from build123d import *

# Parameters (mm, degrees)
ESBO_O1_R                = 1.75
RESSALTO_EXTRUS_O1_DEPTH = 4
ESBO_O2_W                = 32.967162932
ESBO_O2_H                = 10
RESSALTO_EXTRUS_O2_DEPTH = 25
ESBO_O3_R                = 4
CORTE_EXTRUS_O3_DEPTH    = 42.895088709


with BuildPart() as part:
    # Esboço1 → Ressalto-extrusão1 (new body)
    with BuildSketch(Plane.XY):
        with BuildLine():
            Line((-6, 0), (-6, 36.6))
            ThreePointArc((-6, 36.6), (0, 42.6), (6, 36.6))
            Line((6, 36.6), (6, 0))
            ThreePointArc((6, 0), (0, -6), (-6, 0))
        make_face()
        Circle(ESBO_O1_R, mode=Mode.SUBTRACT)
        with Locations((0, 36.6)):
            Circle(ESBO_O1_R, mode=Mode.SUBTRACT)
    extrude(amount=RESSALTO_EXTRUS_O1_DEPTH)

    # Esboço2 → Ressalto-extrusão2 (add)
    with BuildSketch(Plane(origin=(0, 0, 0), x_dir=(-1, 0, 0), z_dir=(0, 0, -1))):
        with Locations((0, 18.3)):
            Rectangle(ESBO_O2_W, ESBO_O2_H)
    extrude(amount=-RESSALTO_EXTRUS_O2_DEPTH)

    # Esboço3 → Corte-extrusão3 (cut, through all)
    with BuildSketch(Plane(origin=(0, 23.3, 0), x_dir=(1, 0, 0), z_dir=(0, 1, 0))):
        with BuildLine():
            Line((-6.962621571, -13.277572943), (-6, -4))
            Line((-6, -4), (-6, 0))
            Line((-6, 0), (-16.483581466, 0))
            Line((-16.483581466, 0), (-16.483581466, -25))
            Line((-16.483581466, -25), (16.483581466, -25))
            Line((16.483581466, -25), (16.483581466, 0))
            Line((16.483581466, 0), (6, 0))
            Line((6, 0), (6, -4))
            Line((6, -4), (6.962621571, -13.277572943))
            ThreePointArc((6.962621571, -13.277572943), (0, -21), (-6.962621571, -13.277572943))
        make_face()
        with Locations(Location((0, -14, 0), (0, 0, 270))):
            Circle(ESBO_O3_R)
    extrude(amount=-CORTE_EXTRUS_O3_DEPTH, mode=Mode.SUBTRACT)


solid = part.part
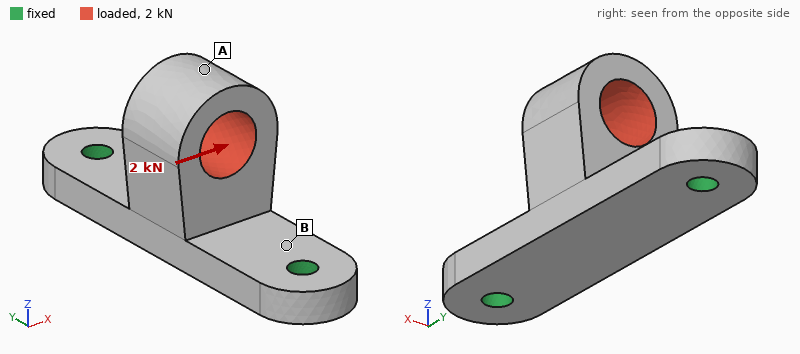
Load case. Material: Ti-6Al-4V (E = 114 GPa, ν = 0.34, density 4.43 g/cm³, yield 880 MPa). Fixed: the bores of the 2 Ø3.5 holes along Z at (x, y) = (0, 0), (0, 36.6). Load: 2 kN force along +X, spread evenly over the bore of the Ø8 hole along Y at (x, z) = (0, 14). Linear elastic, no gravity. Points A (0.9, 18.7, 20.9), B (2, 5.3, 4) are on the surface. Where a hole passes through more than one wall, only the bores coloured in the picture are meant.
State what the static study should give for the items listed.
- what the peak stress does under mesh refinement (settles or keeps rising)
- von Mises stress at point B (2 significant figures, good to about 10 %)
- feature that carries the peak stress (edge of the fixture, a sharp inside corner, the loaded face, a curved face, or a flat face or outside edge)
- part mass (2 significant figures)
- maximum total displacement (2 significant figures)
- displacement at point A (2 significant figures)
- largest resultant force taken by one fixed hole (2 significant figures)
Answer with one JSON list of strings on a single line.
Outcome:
["keeps rising", "380 MPa", "edge of the fixture", "16 g", "0.36 mm", "0.36 mm", "1.0 kN"]
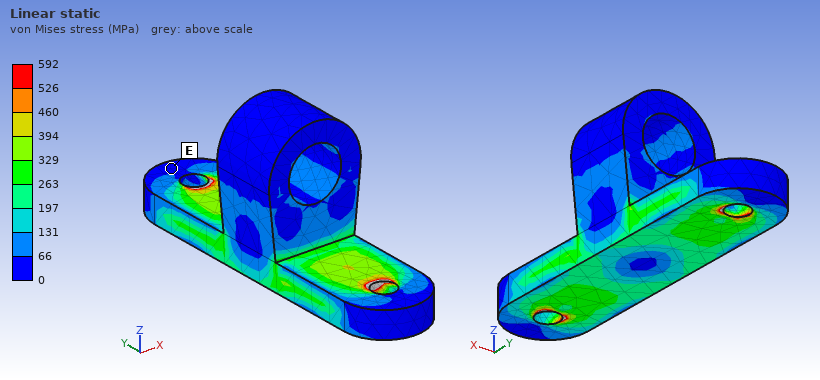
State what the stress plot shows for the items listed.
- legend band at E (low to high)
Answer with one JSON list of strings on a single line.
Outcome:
["0 to 66 MPa"]
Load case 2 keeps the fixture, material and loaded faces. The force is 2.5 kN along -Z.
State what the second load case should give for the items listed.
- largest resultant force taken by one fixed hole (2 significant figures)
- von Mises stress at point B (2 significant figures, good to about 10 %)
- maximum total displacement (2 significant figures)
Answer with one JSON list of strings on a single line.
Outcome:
["1.3 kN", "83 MPa", "60 µm"]
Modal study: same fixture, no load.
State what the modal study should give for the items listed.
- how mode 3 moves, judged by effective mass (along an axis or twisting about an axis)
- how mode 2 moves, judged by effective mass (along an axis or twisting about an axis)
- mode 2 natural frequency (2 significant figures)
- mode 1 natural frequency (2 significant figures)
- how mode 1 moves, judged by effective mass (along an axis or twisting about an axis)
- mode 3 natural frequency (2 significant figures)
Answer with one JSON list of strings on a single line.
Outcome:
["along Y", "along Z", "10 kHz", "5800 Hz", "along X", "12 kHz"]
